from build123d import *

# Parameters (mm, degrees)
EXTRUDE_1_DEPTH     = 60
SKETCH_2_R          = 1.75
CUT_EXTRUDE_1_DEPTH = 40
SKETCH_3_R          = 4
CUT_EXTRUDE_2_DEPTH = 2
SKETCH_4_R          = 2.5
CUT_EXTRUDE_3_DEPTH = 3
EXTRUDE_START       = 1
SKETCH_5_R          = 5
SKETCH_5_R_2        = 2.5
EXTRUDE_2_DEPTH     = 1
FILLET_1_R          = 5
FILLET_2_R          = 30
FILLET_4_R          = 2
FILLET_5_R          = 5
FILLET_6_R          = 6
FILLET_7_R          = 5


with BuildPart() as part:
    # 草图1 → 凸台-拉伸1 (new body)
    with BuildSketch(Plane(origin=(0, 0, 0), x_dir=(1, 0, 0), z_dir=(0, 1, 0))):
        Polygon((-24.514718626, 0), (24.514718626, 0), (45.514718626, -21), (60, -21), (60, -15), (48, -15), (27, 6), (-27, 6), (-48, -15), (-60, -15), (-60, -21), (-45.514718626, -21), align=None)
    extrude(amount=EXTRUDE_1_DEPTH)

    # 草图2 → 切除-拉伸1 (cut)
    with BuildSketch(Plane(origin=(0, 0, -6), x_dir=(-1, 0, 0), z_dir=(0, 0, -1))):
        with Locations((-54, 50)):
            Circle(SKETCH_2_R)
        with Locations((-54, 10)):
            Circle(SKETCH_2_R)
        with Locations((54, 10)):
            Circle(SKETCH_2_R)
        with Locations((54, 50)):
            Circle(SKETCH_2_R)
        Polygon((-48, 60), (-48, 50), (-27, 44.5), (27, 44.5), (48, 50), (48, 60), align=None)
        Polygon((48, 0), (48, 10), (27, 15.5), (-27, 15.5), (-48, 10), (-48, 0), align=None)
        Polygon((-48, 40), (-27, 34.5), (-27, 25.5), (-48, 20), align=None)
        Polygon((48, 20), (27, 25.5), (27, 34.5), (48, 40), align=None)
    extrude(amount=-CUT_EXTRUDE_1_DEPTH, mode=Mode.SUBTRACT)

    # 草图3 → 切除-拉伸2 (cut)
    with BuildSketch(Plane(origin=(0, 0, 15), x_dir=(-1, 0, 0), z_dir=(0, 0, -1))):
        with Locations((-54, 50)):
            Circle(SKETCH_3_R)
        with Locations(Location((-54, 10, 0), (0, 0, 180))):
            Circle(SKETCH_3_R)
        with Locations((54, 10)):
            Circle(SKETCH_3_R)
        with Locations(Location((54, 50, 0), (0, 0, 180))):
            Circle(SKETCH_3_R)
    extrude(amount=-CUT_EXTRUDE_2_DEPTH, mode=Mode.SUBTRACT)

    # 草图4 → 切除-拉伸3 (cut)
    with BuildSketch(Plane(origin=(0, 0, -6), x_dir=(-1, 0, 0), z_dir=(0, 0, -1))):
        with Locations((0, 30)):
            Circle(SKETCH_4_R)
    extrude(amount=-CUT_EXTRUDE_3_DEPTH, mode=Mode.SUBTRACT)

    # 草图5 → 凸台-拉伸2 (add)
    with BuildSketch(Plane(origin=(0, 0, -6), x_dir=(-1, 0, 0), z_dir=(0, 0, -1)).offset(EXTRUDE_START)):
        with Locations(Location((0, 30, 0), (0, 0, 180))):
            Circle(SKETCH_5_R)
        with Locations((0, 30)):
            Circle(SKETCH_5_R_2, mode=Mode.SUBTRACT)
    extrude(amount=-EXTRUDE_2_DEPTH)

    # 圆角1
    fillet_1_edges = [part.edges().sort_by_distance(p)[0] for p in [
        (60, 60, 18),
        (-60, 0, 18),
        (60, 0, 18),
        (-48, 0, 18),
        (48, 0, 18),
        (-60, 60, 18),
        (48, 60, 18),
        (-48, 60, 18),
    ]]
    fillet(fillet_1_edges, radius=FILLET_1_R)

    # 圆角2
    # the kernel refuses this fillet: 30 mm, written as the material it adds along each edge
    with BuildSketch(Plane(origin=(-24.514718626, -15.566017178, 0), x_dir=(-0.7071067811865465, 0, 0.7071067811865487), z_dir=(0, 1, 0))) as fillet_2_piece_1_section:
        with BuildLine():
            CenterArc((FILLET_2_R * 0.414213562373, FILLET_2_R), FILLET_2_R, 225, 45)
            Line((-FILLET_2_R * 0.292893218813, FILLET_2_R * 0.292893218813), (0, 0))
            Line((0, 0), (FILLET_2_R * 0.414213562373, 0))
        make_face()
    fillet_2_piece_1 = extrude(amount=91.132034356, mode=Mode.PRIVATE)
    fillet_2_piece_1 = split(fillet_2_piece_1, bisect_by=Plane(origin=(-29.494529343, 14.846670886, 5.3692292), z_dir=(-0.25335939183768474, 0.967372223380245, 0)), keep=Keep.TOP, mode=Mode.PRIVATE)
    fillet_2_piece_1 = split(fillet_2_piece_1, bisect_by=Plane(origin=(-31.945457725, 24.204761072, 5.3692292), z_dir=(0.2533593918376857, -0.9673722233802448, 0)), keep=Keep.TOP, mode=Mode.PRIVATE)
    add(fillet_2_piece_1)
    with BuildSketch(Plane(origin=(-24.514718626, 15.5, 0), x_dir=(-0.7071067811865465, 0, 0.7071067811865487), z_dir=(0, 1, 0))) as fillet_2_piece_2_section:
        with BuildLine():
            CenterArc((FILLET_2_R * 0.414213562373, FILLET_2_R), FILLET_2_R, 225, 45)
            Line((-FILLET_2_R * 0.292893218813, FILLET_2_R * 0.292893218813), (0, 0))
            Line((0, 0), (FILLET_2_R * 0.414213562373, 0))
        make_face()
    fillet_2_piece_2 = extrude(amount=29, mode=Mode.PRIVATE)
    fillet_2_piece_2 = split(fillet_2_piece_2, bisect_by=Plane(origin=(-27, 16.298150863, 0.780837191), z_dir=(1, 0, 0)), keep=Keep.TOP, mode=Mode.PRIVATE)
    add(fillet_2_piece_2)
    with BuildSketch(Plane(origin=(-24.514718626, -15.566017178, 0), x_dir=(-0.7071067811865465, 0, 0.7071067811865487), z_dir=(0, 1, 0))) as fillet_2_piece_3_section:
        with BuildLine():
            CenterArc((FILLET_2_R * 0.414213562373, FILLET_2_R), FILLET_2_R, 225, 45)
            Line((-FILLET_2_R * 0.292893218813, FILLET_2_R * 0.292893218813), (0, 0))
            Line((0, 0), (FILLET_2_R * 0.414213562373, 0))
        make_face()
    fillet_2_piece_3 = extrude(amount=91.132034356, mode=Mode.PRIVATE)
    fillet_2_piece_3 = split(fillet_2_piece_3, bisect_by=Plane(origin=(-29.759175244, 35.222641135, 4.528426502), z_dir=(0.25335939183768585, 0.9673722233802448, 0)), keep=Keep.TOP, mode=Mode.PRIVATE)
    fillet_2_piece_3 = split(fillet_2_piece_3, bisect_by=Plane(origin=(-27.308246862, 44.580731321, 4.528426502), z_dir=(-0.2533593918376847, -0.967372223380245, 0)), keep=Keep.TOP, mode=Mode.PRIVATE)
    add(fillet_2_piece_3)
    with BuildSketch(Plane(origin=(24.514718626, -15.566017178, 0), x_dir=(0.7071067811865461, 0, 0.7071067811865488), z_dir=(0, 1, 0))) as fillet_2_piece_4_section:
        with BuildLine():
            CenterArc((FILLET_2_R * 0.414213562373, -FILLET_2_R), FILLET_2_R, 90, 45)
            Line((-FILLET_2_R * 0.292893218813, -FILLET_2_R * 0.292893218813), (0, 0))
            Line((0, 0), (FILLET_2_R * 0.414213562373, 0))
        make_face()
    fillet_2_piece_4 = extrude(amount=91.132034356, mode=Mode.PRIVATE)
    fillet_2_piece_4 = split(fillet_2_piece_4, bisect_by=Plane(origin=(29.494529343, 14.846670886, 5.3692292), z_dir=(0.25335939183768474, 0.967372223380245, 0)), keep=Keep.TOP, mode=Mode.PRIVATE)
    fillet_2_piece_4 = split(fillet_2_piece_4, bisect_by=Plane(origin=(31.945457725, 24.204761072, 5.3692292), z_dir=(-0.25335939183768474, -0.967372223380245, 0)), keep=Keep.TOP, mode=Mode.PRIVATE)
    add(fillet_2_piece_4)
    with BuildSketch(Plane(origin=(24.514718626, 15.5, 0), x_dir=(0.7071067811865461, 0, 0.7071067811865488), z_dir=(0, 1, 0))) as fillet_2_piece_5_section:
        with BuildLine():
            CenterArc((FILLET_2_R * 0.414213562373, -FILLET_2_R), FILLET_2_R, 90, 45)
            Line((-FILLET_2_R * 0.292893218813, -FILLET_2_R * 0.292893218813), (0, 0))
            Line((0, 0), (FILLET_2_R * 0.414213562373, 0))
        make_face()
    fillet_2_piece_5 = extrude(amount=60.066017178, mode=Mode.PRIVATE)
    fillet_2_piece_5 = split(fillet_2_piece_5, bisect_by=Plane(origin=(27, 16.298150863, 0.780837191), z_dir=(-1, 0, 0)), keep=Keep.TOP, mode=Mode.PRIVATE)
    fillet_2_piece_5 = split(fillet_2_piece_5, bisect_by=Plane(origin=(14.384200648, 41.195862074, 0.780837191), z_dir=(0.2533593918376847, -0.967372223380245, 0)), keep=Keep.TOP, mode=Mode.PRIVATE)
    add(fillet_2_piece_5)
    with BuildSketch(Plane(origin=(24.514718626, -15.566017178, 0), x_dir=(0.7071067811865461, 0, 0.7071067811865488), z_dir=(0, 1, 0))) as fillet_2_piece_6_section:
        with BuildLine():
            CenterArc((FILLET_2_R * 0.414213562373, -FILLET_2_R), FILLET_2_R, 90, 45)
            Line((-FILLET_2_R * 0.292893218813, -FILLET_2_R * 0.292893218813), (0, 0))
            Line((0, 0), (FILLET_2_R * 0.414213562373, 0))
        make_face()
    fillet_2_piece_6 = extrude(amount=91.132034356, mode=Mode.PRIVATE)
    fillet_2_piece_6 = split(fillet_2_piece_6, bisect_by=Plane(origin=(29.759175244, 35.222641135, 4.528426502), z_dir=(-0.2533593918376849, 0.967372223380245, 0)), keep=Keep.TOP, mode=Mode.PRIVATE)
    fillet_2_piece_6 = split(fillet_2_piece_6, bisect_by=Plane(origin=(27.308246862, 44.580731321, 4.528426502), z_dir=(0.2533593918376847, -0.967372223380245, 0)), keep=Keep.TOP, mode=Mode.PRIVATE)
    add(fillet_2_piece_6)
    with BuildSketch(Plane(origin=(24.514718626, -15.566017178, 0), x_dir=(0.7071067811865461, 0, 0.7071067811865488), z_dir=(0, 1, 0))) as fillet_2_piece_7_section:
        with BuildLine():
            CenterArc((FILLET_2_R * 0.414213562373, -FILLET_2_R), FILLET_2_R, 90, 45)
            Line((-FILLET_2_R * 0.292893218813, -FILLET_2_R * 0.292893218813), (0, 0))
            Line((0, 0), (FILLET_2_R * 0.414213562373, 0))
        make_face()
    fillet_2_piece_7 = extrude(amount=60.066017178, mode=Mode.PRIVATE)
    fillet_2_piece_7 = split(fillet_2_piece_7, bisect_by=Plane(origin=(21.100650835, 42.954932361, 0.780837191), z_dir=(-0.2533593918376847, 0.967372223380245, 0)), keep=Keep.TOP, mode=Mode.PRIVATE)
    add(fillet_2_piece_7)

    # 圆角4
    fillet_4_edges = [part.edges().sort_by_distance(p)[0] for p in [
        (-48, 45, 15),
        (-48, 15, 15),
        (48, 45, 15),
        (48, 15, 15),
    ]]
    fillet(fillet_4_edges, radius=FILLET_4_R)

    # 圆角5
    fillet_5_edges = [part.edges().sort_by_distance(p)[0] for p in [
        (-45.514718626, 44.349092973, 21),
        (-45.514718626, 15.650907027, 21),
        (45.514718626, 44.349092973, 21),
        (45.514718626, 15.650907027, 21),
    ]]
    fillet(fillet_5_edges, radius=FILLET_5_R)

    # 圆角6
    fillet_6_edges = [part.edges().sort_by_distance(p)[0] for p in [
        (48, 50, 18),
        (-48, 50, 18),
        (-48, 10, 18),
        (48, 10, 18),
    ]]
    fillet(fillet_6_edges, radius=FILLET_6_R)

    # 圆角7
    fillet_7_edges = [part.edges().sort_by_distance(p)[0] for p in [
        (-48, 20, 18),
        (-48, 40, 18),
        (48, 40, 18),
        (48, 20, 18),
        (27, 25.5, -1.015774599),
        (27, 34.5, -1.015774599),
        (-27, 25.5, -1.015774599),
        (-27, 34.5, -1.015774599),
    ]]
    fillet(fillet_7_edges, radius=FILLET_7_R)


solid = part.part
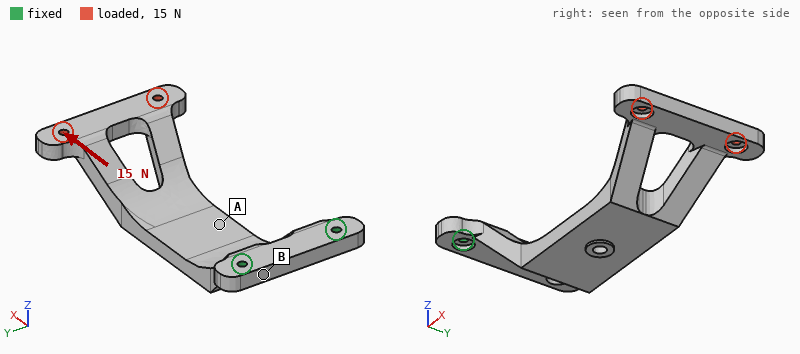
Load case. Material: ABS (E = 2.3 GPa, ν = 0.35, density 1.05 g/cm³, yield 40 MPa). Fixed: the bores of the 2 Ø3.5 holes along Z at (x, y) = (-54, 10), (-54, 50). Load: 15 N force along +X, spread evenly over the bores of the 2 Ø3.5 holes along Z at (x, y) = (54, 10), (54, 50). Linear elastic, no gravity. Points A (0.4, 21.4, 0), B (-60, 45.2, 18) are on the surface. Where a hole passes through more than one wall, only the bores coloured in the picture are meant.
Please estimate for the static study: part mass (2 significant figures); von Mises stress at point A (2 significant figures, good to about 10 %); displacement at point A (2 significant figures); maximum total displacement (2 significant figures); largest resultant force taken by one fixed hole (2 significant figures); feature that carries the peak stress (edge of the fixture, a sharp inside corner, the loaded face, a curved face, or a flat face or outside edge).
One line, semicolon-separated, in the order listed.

27 g; 1.9 MPa; 0.23 mm; 1.3 mm; 7.8 N; a curved face
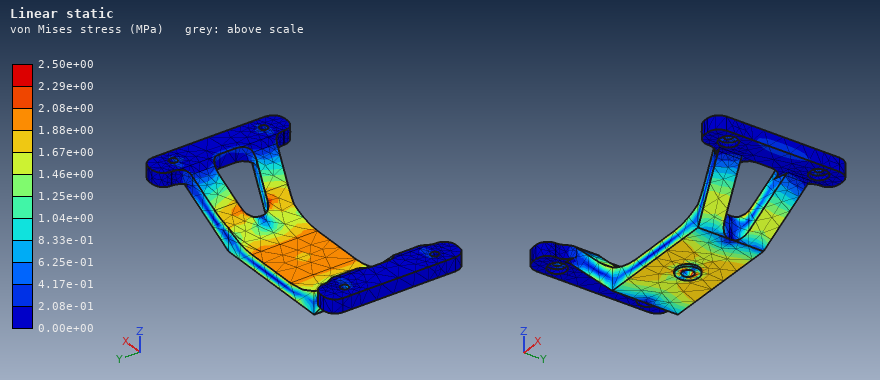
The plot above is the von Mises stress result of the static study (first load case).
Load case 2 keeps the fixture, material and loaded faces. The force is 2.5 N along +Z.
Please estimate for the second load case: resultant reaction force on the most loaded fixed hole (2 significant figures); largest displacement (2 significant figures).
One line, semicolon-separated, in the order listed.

1.6 N; 1.4 mm
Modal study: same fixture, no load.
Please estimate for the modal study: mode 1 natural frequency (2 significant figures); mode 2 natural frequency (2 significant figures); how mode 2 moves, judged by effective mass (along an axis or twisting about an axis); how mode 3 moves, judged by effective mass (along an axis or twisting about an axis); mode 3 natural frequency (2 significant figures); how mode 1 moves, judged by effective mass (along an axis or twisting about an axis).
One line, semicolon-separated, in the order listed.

75 Hz; 180 Hz; along Y; along X; 360 Hz; along Z
